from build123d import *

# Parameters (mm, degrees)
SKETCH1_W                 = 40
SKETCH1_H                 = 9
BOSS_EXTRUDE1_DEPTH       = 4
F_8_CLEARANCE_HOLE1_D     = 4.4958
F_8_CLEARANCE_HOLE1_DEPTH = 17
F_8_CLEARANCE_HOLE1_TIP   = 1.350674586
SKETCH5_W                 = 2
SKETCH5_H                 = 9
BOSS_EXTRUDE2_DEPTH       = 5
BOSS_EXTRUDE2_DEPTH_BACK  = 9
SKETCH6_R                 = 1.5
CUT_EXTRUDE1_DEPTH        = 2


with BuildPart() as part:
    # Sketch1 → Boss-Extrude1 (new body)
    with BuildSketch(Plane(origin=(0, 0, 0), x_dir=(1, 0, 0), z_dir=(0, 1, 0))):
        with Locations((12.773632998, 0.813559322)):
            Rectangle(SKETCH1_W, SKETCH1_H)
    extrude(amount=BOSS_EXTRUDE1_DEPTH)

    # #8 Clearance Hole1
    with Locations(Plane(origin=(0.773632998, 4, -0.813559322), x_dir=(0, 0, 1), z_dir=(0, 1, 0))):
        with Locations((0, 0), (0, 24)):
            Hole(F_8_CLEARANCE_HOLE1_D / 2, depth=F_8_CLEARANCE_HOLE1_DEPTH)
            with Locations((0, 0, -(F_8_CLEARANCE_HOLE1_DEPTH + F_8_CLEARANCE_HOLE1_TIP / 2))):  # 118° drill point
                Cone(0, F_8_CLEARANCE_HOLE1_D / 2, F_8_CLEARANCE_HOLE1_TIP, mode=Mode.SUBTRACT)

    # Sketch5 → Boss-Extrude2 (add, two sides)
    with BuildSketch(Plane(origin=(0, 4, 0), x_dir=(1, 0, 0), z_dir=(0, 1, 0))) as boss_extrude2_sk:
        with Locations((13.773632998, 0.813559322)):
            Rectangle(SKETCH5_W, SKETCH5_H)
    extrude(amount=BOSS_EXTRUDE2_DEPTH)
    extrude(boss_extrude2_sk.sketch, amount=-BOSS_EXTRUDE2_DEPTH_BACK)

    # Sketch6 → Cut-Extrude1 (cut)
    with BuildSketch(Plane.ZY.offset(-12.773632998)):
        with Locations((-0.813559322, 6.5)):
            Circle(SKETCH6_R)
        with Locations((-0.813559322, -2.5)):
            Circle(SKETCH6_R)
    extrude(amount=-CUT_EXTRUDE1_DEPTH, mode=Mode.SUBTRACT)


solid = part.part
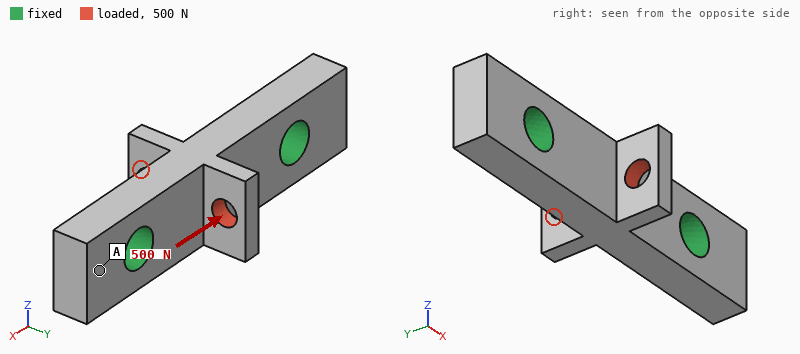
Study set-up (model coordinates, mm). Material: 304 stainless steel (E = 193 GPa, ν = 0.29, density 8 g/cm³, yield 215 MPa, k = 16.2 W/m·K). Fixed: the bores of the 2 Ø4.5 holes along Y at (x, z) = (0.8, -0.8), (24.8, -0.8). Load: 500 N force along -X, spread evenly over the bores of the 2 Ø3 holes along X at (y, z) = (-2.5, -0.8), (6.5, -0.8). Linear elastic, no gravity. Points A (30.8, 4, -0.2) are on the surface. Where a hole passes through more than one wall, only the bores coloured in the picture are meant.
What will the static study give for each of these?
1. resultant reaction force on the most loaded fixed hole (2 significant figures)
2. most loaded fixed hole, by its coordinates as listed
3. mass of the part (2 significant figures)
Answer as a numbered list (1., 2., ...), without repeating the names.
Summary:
1. 270 N
2. (24.8, -0.8)
3. 12 g
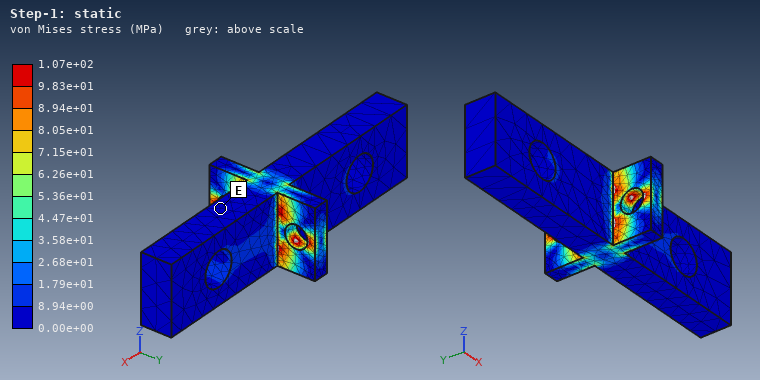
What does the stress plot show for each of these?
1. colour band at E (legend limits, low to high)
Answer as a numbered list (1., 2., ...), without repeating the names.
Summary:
1. 0.00e+00 to 8.94e+00 MPa
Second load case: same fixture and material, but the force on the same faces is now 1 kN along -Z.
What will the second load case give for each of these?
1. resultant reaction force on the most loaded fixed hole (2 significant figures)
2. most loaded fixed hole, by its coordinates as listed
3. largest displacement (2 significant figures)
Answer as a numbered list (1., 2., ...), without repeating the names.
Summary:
1. 560 N
2. (24.8, -0.8)
3. 8.0 µm
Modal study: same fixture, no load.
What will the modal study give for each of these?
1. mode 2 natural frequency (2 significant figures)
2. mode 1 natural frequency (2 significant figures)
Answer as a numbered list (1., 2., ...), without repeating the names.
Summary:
1. 32 kHz
2. 31 kHz
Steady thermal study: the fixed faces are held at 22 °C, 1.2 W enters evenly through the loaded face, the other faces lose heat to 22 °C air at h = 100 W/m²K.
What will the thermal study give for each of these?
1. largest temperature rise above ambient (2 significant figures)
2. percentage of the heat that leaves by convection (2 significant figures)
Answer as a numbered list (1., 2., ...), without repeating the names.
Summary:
1. 16 K
2. 36 %
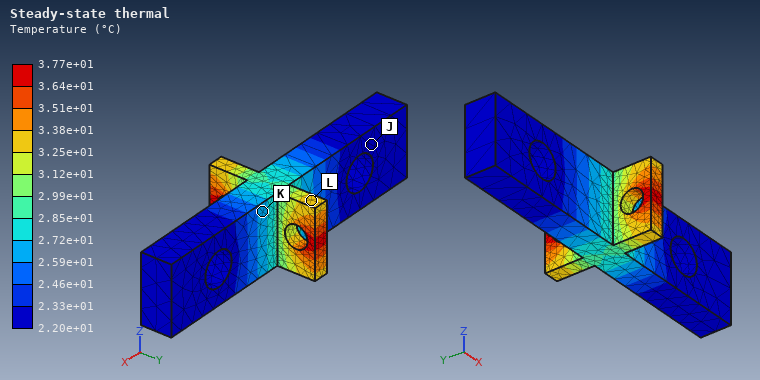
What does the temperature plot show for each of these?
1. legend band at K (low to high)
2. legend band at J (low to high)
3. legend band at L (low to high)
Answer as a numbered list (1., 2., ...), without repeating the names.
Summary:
1. 2.59e+01 to 2.72e+01 °C
2. 2.20e+01 to 2.33e+01 °C
3. 3.25e+01 to 3.38e+01 °C
